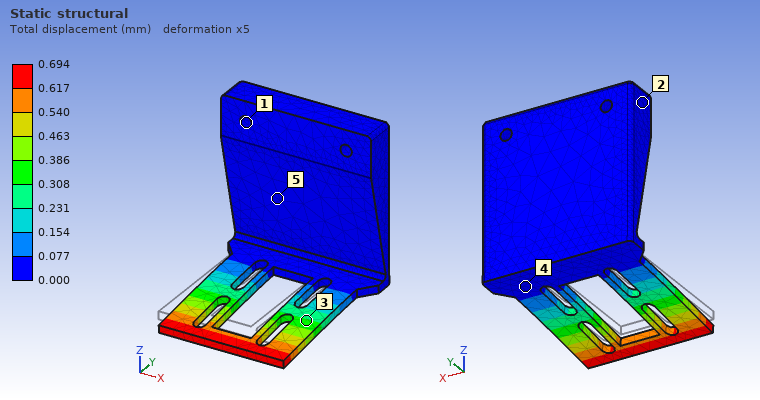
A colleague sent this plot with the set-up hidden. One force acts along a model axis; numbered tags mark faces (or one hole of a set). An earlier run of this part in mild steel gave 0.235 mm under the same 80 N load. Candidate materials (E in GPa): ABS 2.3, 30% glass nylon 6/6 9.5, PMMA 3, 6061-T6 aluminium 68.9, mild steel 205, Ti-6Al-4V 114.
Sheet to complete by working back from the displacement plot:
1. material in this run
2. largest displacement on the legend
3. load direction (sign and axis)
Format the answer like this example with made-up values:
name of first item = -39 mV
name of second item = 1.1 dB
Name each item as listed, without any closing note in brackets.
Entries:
material in this run = 6061-T6 aluminium
largest displacement on the legend = 0.694 mm
load direction = -Z
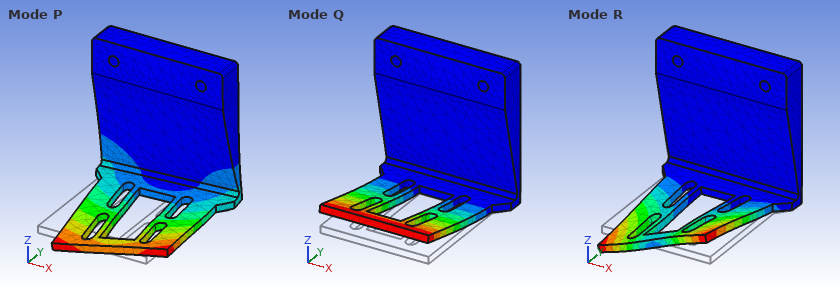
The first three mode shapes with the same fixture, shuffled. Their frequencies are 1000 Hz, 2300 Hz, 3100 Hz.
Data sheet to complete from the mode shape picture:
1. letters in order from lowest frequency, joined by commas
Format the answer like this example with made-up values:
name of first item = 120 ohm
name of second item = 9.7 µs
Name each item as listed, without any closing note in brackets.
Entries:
letters in order from lowest frequency, joined by commas = Q, R, P
